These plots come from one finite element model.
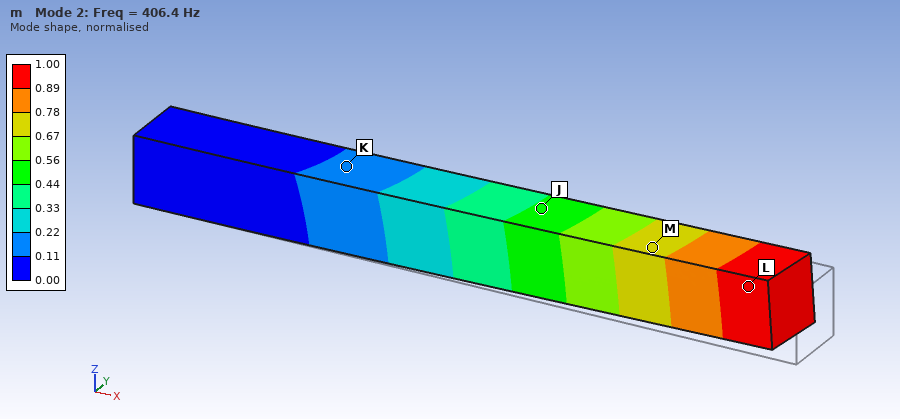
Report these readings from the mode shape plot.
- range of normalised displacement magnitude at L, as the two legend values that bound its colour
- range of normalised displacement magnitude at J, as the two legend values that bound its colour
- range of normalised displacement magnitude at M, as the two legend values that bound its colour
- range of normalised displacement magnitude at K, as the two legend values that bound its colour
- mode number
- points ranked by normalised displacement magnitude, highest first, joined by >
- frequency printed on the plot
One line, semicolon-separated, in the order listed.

0.89 to 1.00; 0.44 to 0.56; 0.67 to 0.78; 0.11 to 0.22; 2; L > M > J > K; 406.4 Hz
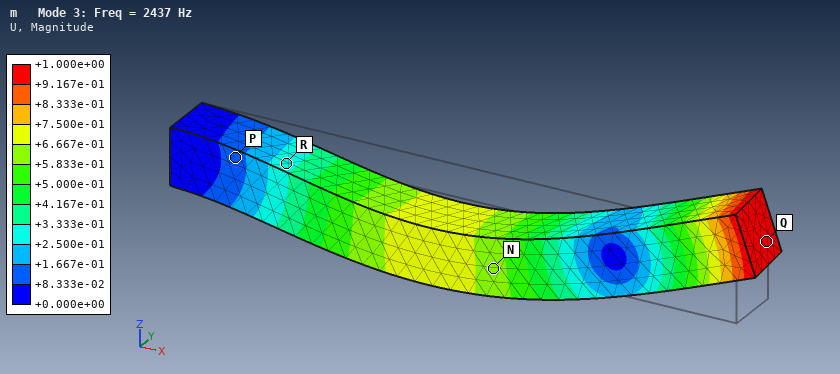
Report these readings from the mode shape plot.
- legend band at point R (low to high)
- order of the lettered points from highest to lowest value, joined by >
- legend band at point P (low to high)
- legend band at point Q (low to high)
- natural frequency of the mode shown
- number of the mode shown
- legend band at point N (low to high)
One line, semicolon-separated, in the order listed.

+2.500e-01 to +3.333e-01; Q > N > R > P; +8.333e-02 to +1.667e-01; +9.167e-01 to +1.000e+00; 2437 Hz; 3; +5.833e-01 to +6.667e-01
